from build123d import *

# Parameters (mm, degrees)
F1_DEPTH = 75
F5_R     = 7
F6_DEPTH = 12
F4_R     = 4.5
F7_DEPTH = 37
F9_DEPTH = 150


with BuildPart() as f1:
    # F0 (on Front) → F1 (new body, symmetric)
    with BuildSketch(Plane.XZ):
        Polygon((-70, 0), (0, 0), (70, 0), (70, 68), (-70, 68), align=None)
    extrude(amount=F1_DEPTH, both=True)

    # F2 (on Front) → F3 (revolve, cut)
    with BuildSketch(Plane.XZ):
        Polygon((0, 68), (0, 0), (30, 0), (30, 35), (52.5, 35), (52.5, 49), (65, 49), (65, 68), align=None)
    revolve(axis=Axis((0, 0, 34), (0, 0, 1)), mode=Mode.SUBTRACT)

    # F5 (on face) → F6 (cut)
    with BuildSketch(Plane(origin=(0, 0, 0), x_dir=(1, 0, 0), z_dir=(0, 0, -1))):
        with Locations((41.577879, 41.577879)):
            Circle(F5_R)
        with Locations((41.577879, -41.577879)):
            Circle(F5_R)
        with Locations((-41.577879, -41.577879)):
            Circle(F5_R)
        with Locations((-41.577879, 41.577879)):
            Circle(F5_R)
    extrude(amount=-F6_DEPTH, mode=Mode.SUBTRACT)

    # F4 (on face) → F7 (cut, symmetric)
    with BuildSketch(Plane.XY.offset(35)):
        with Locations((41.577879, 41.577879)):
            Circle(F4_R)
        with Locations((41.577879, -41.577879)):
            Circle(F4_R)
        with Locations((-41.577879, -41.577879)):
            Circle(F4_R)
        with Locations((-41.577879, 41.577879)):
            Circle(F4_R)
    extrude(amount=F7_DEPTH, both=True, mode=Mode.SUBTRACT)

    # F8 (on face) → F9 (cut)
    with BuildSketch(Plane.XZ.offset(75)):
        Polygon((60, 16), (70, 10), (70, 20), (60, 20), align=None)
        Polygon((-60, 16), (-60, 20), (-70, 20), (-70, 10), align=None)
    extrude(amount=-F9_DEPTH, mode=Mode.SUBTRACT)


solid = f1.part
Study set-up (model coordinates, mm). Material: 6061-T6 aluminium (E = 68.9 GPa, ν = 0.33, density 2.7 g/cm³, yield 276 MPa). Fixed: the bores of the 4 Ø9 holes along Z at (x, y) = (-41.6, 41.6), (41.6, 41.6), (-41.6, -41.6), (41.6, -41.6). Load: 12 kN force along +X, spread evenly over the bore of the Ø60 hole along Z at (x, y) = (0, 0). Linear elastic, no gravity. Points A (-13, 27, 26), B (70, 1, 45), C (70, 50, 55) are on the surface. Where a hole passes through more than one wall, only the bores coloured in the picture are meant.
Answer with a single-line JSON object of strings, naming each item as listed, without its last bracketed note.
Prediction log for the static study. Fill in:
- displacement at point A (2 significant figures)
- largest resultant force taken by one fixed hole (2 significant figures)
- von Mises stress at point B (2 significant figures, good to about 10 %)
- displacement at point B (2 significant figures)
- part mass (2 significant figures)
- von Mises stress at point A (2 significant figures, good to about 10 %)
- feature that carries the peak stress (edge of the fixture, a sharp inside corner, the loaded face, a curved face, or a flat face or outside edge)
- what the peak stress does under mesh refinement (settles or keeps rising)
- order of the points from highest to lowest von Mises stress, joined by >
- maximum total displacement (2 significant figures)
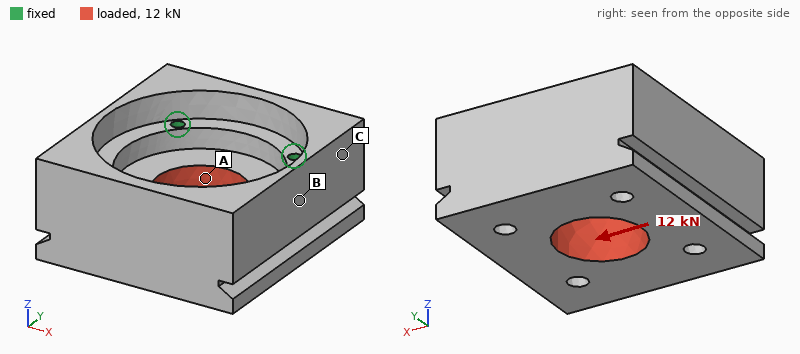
{"displacement at point A": "1.5 µm", "largest resultant force taken by one fixed hole": "3.1 kN", "von Mises stress at point B": "1.4 MPa", "displacement at point B": "1.0 µm", "part mass": "2.5 kg", "von Mises stress at point A": "3.3 MPa", "feature that carries the peak stress": "edge of the fixture", "what the peak stress does under mesh refinement": "keeps rising", "order of the points from highest to lowest von Mises stress, joined by >": "A > B > C", "maximum total displacement": "3.0 µm"}
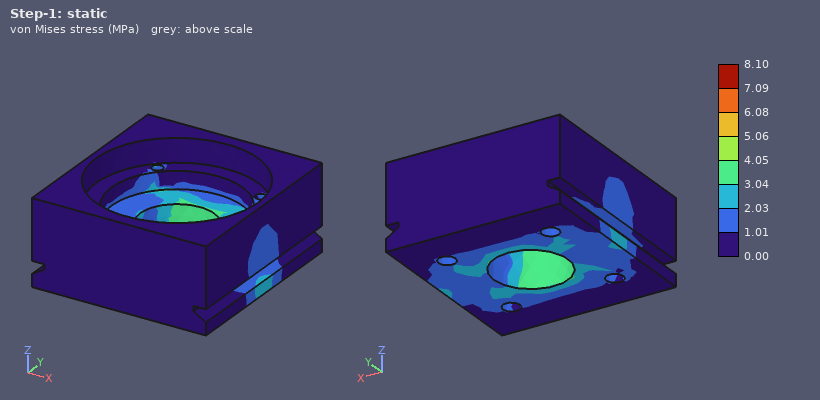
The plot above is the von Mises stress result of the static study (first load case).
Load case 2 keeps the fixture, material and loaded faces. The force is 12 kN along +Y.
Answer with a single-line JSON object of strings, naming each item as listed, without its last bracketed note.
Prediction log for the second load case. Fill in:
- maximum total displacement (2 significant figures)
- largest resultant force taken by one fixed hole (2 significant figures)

{"maximum total displacement": "2.7 µm", "largest resultant force taken by one fixed hole": "3.0 kN"}
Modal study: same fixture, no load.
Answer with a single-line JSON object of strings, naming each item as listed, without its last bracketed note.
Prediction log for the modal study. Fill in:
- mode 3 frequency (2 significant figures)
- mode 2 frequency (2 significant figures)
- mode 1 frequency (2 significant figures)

{"mode 3 frequency": "9600 Hz", "mode 2 frequency": "8600 Hz", "mode 1 frequency": "8600 Hz"}
